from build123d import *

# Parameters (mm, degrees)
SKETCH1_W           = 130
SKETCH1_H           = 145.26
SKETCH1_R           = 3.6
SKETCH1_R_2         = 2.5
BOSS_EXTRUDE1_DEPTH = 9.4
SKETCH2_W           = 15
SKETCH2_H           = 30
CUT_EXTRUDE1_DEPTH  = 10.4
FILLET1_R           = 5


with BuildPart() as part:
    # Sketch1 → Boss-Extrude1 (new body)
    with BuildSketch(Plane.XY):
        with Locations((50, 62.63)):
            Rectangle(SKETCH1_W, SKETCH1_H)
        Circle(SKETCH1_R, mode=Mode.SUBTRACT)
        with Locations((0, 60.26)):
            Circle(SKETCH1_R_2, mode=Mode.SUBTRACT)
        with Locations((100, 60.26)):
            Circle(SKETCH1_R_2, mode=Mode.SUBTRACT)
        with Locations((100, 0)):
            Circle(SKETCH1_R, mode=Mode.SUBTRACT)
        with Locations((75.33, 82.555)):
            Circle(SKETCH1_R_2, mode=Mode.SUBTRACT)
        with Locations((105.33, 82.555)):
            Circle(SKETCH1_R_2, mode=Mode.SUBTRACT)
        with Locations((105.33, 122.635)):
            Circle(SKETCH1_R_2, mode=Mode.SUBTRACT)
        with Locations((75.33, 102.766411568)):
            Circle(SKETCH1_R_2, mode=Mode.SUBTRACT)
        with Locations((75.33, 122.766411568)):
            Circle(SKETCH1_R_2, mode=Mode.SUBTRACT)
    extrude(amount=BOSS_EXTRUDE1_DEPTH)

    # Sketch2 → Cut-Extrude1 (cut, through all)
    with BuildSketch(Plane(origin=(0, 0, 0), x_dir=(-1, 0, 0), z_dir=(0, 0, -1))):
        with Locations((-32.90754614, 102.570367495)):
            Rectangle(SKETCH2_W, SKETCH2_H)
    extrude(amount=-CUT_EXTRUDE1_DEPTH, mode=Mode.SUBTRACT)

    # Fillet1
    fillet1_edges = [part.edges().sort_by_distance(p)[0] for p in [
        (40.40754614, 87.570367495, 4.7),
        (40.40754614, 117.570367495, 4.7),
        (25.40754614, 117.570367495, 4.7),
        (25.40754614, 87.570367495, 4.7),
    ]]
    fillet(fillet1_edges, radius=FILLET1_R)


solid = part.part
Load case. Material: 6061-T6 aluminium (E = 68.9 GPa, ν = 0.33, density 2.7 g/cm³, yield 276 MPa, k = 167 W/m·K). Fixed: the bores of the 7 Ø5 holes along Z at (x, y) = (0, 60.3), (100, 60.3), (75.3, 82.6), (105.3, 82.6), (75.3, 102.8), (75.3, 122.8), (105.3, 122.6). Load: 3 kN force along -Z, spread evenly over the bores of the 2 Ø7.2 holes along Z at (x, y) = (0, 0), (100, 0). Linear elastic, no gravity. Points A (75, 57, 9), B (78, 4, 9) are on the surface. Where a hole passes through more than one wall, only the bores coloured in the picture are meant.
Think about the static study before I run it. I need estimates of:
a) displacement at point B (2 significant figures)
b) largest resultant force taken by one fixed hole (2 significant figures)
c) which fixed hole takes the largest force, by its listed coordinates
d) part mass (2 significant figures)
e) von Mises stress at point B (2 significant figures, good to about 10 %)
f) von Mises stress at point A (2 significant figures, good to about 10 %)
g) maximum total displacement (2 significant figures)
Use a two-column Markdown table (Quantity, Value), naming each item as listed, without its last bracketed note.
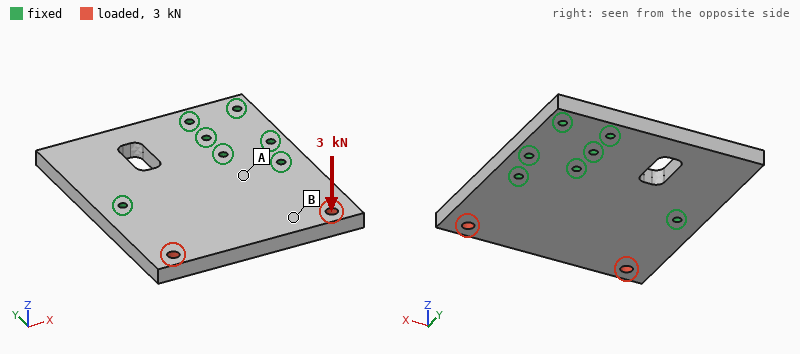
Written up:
| Quantity | Value |
|---|---|
| displacement at point B | 0.44 mm |
| largest resultant force taken by one fixed hole | 3.3 kN |
| which fixed hole takes the largest force, by its listed coordinates | (100, 60.3) |
| part mass | 460 g |
| von Mises stress at point B | 20 MPa |
| von Mises stress at point A | 58 MPa |
| maximum total displacement | 0.62 mm |
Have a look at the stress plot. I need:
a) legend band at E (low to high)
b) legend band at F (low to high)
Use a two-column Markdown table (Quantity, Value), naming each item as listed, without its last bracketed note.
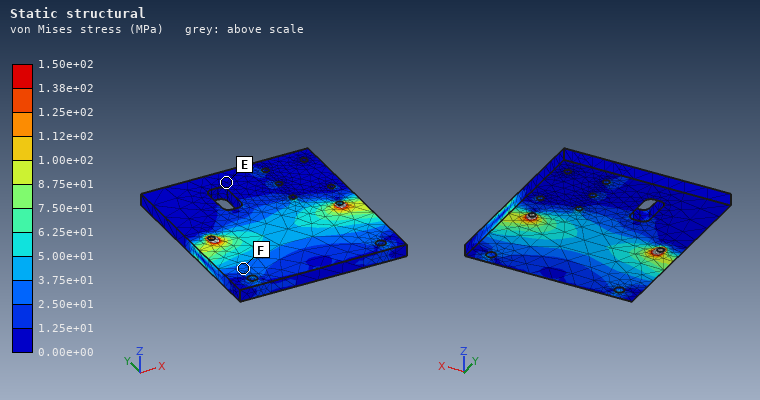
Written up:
| Quantity | Value |
|---|---|
| legend band at E | 0.00e+00 to 1.25e+01 MPa |
| legend band at F | 2.50e+01 to 3.75e+01 MPa |
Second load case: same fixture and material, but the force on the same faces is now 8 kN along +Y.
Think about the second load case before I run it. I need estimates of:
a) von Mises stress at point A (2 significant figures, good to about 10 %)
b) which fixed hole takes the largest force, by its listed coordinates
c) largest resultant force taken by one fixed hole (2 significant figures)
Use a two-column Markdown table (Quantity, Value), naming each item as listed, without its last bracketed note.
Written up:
| Quantity | Value |
|---|---|
| von Mises stress at point A | 4.4 MPa |
| which fixed hole takes the largest force, by its listed coordinates | (0, 60.3) |
| largest resultant force taken by one fixed hole | 3.4 kN |
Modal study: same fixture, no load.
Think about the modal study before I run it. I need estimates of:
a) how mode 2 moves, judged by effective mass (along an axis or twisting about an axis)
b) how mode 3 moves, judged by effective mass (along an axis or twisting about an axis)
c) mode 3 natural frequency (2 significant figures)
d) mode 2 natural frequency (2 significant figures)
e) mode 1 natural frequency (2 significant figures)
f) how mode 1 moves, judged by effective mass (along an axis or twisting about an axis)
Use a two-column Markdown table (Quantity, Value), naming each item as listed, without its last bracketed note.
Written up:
| Quantity | Value |
|---|---|
| how mode 2 moves, judged by effective mass | along Z |
| how mode 3 moves, judged by effective mass | twisting about Y |
| mode 3 natural frequency | 2400 Hz |
| mode 2 natural frequency | 2100 Hz |
| mode 1 natural frequency | 1200 Hz |
| how mode 1 moves, judged by effective mass | along Z |
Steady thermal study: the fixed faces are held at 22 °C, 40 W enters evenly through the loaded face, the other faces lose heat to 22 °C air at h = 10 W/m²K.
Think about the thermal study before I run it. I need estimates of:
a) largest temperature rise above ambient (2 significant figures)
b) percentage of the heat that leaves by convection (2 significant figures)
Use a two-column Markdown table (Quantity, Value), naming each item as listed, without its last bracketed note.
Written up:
| Quantity | Value |
|---|---|
| largest temperature rise above ambient | 19 K |
| percentage of the heat that leaves by convection | 5.3 % |
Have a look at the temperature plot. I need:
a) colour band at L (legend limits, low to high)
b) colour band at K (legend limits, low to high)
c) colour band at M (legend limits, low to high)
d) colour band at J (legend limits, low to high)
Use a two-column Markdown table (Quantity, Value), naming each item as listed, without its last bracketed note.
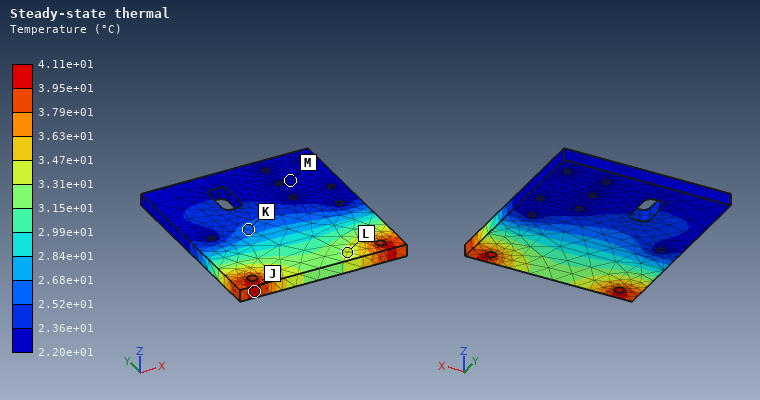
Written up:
| Quantity | Value |
|---|---|
| colour band at L | 3.31e+01 to 3.47e+01 °C |
| colour band at K | 2.52e+01 to 2.68e+01 °C |
| colour band at M | 2.20e+01 to 2.36e+01 °C |
| colour band at J | 3.95e+01 to 4.11e+01 °C |
